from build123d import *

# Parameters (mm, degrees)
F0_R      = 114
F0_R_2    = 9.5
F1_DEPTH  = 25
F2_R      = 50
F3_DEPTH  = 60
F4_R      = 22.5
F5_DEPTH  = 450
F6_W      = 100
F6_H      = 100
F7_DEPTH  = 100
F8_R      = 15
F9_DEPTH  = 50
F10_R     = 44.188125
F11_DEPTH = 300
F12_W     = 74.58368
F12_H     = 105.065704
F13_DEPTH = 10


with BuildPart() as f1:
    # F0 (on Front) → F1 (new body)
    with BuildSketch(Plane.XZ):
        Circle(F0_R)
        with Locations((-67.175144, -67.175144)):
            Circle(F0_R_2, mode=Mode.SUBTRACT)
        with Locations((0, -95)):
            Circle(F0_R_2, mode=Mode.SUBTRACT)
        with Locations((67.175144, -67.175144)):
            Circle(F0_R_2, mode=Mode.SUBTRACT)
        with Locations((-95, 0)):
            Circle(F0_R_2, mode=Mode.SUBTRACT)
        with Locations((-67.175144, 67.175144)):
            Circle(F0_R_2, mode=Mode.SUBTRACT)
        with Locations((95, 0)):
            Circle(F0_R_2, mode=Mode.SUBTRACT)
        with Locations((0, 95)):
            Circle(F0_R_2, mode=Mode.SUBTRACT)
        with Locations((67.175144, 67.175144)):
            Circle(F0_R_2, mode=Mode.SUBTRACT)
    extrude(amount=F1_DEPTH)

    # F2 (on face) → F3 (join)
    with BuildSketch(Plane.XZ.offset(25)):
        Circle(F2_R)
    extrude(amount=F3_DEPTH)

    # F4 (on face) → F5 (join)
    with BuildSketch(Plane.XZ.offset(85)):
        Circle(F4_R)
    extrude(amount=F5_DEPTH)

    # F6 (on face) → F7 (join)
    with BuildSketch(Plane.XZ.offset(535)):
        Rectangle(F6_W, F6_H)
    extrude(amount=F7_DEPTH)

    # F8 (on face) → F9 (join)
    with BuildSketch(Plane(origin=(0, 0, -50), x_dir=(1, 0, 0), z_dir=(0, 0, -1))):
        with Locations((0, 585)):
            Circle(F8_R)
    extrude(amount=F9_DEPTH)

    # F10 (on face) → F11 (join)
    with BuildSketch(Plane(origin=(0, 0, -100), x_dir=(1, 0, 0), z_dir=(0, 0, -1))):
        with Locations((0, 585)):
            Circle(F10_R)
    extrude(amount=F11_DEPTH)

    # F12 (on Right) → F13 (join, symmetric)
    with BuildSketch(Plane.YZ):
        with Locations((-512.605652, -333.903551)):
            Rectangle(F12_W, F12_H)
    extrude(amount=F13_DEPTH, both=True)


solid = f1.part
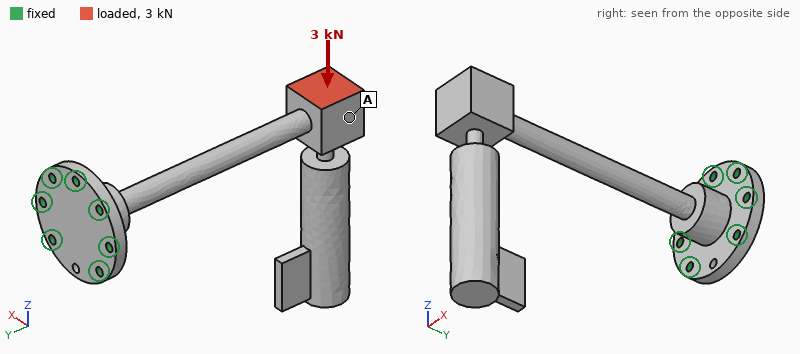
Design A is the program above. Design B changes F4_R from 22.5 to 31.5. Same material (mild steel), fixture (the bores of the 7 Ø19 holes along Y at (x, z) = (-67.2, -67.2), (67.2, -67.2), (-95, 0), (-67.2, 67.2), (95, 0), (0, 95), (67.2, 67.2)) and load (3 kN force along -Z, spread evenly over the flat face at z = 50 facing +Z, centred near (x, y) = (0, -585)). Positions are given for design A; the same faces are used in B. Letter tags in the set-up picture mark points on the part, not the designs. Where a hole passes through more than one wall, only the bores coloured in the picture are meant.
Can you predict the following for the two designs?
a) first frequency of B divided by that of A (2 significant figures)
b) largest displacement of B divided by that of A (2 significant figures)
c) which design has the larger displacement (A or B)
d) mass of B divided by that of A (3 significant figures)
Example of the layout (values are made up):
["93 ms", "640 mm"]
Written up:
["1.7", "0.28", "A", "1.13"]
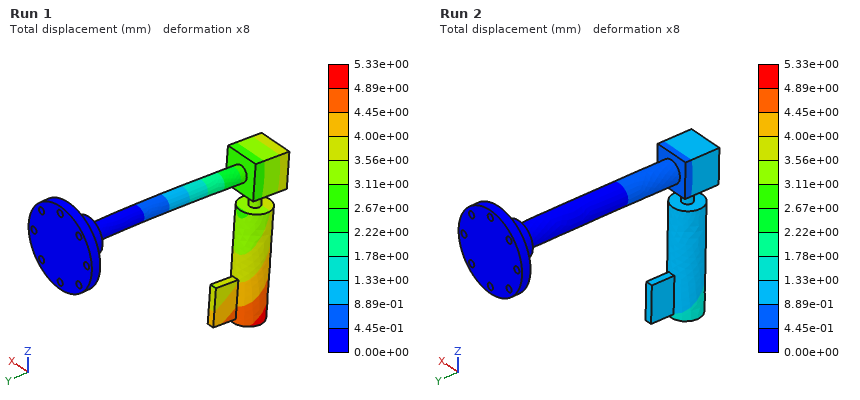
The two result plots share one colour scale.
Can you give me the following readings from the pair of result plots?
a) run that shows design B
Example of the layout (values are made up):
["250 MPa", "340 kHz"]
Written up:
["Run 2"]
